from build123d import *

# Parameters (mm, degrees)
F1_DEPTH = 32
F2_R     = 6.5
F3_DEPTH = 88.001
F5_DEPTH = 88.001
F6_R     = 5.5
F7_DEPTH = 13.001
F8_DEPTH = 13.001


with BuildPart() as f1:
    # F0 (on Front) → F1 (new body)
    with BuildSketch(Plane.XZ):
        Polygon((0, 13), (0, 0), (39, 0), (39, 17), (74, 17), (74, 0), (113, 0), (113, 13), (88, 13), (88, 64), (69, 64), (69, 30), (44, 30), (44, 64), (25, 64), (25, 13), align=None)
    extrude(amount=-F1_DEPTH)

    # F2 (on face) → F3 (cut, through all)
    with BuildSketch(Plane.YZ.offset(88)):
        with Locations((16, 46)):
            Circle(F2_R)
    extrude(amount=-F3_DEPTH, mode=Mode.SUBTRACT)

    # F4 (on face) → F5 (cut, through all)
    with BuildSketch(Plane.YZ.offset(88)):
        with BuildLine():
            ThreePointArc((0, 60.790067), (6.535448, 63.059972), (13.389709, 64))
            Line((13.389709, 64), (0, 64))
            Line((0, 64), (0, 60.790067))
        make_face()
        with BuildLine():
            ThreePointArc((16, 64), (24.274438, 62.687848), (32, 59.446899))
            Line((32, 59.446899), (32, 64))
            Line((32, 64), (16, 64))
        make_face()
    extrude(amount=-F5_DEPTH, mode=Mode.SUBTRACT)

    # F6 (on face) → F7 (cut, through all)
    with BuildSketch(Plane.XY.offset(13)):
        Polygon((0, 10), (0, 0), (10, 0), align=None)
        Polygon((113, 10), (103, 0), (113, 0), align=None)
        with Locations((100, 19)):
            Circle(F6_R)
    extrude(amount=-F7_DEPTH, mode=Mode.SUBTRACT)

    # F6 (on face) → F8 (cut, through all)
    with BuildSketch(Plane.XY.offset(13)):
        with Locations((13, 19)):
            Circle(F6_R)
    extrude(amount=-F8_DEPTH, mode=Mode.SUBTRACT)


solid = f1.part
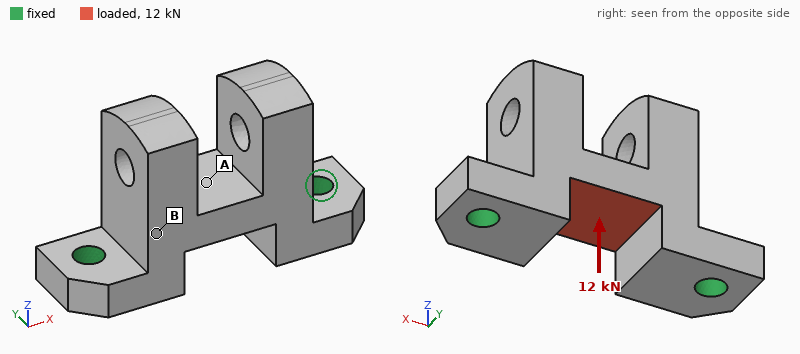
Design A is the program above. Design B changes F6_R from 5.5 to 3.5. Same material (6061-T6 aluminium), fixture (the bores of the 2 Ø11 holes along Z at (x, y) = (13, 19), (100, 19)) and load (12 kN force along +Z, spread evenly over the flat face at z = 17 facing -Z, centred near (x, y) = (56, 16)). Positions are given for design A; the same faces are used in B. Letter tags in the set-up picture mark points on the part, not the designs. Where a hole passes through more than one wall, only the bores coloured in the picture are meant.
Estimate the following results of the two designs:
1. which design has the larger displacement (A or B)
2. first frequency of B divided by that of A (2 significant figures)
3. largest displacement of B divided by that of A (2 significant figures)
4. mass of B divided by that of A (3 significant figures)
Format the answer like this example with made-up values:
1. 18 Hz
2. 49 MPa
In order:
1. B
2. 0.86
3. 1.2
4. 1.02
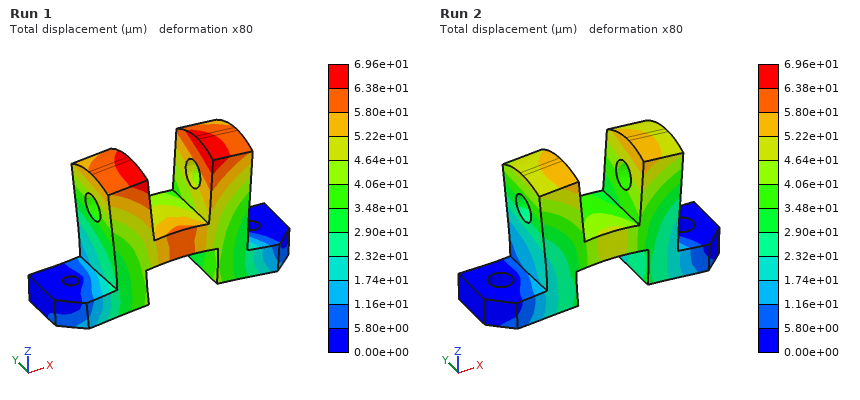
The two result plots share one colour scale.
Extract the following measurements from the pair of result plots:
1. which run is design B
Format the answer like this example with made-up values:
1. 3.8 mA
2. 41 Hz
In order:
1. Run 1
